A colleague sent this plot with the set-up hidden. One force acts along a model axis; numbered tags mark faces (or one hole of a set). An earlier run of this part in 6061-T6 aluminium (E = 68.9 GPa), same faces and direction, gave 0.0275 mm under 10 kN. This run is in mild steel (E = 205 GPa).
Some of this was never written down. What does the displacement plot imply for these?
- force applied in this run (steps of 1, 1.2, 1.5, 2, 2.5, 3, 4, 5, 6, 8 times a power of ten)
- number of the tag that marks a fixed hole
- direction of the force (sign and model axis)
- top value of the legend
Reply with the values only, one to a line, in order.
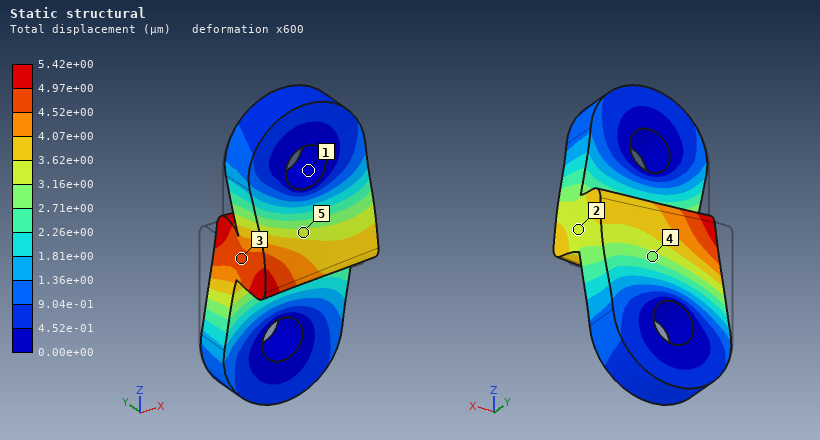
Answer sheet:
6 kN
1
+X
5.42e+00 µm
